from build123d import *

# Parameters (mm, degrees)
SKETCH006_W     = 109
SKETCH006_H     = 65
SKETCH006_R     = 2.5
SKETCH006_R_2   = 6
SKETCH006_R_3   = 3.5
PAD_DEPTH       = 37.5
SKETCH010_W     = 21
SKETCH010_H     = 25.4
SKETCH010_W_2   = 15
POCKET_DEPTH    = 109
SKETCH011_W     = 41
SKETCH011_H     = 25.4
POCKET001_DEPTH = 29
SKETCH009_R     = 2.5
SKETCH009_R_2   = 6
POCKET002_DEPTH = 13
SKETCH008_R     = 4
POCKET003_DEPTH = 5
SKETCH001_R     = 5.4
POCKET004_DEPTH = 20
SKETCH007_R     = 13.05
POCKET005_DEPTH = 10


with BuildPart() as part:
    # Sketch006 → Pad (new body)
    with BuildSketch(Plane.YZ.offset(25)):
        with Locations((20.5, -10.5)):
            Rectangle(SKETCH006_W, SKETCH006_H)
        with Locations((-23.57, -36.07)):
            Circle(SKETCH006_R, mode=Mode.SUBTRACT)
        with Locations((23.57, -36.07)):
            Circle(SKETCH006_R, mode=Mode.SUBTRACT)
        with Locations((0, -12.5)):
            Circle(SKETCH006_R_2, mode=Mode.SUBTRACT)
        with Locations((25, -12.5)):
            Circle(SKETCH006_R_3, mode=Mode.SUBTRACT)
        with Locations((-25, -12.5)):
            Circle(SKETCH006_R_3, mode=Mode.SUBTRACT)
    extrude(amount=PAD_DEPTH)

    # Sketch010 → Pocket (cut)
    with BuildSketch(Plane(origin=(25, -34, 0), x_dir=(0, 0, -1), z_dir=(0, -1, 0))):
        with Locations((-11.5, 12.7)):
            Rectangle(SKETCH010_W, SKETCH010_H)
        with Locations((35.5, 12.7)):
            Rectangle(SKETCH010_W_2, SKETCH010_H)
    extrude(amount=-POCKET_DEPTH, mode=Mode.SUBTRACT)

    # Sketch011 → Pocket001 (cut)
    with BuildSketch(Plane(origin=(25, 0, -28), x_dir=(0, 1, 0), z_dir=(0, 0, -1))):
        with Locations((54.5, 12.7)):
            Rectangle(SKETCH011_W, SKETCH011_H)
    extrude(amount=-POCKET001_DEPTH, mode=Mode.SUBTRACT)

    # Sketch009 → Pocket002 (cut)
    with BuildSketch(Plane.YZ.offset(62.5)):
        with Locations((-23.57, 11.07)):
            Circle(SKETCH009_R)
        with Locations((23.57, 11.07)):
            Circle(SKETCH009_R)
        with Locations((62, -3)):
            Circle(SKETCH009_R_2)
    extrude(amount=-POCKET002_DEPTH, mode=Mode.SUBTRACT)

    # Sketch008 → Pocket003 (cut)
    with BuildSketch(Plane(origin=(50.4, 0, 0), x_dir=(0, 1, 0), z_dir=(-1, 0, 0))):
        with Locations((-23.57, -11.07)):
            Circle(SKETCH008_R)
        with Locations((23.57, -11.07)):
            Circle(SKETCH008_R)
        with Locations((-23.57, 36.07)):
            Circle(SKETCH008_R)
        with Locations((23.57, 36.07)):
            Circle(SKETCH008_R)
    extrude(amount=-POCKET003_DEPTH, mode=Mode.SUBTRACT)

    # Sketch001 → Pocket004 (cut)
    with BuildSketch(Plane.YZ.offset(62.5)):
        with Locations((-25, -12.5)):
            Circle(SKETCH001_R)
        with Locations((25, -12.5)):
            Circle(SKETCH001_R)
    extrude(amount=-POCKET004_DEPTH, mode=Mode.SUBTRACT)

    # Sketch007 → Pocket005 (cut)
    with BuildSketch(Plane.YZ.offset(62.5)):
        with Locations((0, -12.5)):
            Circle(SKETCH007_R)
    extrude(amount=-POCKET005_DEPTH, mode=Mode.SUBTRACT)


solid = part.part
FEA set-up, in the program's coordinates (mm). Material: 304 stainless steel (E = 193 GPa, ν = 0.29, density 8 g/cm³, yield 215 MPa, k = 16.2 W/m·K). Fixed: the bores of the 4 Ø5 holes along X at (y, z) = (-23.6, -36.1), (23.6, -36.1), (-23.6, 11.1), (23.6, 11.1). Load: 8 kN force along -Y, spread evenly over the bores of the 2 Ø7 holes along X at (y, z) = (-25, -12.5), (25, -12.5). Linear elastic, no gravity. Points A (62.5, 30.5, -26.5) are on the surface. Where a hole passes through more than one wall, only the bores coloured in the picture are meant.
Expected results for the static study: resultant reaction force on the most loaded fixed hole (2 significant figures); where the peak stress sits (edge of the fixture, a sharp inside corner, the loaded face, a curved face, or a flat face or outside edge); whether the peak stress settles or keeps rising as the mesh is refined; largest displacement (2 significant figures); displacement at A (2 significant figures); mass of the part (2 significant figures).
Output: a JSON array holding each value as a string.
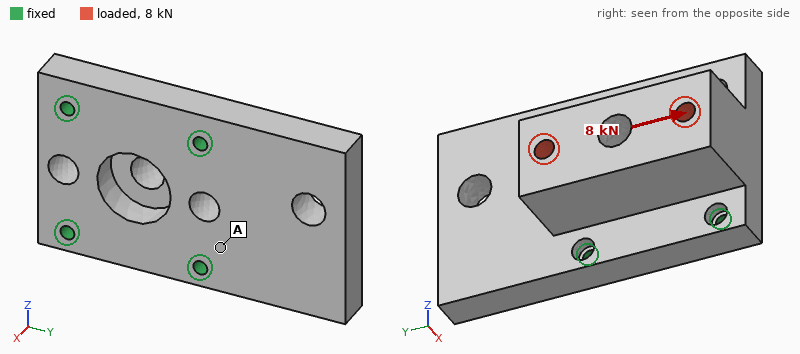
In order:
["3.2 kN", "edge of the fixture", "keeps rising", "12 µm", "3.0 µm", "960 g"]
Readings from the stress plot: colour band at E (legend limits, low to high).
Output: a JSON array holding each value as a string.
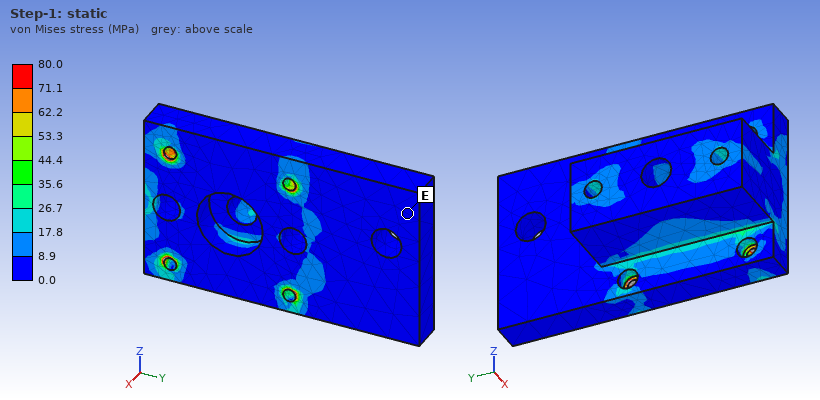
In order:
["0.0 to 8.9 MPa"]
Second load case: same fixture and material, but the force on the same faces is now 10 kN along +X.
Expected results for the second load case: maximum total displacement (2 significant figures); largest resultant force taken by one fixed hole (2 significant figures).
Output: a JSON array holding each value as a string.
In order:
["5.8 µm", "3.0 kN"]
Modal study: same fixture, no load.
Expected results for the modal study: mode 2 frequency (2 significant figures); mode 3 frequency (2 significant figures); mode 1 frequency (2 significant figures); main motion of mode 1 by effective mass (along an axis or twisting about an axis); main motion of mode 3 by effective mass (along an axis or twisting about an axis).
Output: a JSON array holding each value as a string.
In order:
["6200 Hz", "9400 Hz", "3300 Hz", "along X", "along Z"]
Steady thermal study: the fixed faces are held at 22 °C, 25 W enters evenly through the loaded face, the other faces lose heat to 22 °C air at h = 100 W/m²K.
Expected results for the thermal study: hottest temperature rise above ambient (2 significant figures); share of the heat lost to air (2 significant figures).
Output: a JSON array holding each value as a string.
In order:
["28 K", "71 %"]
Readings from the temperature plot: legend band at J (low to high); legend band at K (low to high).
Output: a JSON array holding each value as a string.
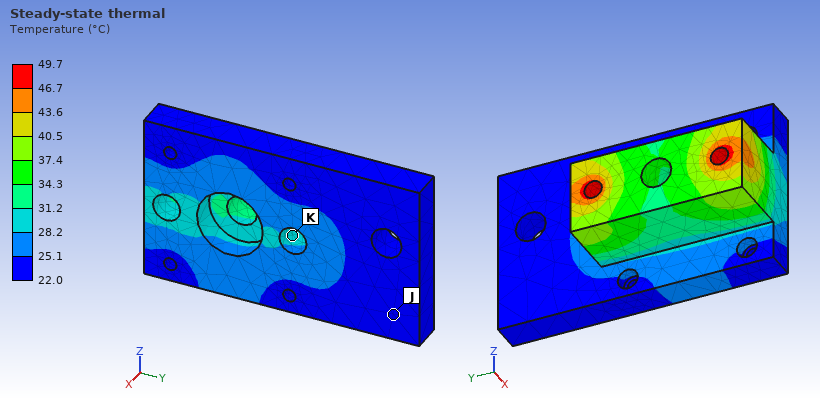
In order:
["22.0 to 25.1 °C", "28.2 to 31.2 °C"]
